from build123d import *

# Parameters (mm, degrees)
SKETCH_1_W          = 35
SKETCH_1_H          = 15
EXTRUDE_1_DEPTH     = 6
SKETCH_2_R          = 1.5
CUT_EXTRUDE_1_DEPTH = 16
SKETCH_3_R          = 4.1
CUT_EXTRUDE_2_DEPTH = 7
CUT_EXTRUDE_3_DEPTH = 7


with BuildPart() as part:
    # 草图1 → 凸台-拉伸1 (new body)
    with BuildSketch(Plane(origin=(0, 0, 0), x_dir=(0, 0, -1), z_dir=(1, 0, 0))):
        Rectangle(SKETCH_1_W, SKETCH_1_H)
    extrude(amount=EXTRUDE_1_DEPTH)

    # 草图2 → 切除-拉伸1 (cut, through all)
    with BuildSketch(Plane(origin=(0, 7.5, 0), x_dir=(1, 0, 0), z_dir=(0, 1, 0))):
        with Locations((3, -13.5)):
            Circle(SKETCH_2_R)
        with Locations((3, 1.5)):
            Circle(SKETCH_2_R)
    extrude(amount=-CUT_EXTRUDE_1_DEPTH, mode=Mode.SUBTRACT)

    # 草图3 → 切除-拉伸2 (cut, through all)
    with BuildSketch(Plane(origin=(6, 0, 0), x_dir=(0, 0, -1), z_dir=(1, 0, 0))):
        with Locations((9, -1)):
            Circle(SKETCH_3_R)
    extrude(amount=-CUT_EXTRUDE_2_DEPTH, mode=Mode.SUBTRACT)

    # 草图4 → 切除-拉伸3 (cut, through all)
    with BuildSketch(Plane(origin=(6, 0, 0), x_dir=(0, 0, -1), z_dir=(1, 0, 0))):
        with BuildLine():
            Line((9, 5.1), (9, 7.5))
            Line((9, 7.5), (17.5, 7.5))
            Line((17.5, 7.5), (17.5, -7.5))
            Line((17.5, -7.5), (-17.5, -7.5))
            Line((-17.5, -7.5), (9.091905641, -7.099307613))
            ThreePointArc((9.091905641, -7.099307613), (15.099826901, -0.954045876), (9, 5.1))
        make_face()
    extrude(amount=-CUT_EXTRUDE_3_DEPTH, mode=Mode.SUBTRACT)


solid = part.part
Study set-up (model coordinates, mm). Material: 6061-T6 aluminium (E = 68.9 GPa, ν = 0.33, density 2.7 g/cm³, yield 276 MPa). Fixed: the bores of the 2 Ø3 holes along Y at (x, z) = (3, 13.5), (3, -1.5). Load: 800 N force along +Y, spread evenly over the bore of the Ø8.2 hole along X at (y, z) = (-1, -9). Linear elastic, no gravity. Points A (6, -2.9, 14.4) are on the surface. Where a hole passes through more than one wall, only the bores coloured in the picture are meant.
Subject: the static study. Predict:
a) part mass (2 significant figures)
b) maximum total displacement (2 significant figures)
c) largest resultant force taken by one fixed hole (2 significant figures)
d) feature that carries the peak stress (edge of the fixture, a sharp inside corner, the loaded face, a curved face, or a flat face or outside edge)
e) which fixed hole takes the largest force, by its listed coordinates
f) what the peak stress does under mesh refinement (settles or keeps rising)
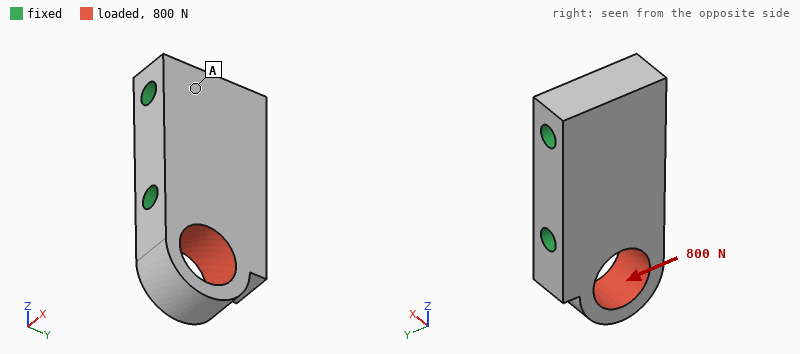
5.9 g
21 µm
810 N
edge of the fixture
(3, -1.5)
keeps rising
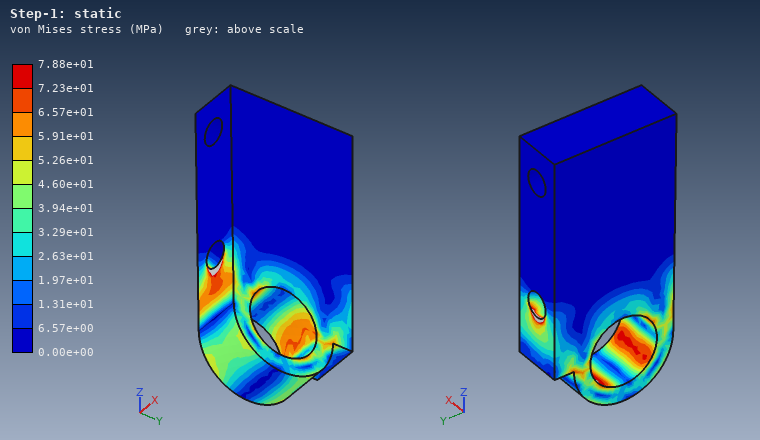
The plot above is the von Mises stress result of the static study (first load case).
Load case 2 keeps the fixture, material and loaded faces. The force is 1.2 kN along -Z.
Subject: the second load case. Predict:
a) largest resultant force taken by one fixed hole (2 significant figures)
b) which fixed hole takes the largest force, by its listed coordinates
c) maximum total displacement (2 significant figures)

1.2 kN
(3, -1.5)
9.0 µm
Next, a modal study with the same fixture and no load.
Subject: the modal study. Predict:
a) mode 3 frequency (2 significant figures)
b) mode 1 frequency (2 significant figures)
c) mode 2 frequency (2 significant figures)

49 kHz
27 kHz
34 kHz
